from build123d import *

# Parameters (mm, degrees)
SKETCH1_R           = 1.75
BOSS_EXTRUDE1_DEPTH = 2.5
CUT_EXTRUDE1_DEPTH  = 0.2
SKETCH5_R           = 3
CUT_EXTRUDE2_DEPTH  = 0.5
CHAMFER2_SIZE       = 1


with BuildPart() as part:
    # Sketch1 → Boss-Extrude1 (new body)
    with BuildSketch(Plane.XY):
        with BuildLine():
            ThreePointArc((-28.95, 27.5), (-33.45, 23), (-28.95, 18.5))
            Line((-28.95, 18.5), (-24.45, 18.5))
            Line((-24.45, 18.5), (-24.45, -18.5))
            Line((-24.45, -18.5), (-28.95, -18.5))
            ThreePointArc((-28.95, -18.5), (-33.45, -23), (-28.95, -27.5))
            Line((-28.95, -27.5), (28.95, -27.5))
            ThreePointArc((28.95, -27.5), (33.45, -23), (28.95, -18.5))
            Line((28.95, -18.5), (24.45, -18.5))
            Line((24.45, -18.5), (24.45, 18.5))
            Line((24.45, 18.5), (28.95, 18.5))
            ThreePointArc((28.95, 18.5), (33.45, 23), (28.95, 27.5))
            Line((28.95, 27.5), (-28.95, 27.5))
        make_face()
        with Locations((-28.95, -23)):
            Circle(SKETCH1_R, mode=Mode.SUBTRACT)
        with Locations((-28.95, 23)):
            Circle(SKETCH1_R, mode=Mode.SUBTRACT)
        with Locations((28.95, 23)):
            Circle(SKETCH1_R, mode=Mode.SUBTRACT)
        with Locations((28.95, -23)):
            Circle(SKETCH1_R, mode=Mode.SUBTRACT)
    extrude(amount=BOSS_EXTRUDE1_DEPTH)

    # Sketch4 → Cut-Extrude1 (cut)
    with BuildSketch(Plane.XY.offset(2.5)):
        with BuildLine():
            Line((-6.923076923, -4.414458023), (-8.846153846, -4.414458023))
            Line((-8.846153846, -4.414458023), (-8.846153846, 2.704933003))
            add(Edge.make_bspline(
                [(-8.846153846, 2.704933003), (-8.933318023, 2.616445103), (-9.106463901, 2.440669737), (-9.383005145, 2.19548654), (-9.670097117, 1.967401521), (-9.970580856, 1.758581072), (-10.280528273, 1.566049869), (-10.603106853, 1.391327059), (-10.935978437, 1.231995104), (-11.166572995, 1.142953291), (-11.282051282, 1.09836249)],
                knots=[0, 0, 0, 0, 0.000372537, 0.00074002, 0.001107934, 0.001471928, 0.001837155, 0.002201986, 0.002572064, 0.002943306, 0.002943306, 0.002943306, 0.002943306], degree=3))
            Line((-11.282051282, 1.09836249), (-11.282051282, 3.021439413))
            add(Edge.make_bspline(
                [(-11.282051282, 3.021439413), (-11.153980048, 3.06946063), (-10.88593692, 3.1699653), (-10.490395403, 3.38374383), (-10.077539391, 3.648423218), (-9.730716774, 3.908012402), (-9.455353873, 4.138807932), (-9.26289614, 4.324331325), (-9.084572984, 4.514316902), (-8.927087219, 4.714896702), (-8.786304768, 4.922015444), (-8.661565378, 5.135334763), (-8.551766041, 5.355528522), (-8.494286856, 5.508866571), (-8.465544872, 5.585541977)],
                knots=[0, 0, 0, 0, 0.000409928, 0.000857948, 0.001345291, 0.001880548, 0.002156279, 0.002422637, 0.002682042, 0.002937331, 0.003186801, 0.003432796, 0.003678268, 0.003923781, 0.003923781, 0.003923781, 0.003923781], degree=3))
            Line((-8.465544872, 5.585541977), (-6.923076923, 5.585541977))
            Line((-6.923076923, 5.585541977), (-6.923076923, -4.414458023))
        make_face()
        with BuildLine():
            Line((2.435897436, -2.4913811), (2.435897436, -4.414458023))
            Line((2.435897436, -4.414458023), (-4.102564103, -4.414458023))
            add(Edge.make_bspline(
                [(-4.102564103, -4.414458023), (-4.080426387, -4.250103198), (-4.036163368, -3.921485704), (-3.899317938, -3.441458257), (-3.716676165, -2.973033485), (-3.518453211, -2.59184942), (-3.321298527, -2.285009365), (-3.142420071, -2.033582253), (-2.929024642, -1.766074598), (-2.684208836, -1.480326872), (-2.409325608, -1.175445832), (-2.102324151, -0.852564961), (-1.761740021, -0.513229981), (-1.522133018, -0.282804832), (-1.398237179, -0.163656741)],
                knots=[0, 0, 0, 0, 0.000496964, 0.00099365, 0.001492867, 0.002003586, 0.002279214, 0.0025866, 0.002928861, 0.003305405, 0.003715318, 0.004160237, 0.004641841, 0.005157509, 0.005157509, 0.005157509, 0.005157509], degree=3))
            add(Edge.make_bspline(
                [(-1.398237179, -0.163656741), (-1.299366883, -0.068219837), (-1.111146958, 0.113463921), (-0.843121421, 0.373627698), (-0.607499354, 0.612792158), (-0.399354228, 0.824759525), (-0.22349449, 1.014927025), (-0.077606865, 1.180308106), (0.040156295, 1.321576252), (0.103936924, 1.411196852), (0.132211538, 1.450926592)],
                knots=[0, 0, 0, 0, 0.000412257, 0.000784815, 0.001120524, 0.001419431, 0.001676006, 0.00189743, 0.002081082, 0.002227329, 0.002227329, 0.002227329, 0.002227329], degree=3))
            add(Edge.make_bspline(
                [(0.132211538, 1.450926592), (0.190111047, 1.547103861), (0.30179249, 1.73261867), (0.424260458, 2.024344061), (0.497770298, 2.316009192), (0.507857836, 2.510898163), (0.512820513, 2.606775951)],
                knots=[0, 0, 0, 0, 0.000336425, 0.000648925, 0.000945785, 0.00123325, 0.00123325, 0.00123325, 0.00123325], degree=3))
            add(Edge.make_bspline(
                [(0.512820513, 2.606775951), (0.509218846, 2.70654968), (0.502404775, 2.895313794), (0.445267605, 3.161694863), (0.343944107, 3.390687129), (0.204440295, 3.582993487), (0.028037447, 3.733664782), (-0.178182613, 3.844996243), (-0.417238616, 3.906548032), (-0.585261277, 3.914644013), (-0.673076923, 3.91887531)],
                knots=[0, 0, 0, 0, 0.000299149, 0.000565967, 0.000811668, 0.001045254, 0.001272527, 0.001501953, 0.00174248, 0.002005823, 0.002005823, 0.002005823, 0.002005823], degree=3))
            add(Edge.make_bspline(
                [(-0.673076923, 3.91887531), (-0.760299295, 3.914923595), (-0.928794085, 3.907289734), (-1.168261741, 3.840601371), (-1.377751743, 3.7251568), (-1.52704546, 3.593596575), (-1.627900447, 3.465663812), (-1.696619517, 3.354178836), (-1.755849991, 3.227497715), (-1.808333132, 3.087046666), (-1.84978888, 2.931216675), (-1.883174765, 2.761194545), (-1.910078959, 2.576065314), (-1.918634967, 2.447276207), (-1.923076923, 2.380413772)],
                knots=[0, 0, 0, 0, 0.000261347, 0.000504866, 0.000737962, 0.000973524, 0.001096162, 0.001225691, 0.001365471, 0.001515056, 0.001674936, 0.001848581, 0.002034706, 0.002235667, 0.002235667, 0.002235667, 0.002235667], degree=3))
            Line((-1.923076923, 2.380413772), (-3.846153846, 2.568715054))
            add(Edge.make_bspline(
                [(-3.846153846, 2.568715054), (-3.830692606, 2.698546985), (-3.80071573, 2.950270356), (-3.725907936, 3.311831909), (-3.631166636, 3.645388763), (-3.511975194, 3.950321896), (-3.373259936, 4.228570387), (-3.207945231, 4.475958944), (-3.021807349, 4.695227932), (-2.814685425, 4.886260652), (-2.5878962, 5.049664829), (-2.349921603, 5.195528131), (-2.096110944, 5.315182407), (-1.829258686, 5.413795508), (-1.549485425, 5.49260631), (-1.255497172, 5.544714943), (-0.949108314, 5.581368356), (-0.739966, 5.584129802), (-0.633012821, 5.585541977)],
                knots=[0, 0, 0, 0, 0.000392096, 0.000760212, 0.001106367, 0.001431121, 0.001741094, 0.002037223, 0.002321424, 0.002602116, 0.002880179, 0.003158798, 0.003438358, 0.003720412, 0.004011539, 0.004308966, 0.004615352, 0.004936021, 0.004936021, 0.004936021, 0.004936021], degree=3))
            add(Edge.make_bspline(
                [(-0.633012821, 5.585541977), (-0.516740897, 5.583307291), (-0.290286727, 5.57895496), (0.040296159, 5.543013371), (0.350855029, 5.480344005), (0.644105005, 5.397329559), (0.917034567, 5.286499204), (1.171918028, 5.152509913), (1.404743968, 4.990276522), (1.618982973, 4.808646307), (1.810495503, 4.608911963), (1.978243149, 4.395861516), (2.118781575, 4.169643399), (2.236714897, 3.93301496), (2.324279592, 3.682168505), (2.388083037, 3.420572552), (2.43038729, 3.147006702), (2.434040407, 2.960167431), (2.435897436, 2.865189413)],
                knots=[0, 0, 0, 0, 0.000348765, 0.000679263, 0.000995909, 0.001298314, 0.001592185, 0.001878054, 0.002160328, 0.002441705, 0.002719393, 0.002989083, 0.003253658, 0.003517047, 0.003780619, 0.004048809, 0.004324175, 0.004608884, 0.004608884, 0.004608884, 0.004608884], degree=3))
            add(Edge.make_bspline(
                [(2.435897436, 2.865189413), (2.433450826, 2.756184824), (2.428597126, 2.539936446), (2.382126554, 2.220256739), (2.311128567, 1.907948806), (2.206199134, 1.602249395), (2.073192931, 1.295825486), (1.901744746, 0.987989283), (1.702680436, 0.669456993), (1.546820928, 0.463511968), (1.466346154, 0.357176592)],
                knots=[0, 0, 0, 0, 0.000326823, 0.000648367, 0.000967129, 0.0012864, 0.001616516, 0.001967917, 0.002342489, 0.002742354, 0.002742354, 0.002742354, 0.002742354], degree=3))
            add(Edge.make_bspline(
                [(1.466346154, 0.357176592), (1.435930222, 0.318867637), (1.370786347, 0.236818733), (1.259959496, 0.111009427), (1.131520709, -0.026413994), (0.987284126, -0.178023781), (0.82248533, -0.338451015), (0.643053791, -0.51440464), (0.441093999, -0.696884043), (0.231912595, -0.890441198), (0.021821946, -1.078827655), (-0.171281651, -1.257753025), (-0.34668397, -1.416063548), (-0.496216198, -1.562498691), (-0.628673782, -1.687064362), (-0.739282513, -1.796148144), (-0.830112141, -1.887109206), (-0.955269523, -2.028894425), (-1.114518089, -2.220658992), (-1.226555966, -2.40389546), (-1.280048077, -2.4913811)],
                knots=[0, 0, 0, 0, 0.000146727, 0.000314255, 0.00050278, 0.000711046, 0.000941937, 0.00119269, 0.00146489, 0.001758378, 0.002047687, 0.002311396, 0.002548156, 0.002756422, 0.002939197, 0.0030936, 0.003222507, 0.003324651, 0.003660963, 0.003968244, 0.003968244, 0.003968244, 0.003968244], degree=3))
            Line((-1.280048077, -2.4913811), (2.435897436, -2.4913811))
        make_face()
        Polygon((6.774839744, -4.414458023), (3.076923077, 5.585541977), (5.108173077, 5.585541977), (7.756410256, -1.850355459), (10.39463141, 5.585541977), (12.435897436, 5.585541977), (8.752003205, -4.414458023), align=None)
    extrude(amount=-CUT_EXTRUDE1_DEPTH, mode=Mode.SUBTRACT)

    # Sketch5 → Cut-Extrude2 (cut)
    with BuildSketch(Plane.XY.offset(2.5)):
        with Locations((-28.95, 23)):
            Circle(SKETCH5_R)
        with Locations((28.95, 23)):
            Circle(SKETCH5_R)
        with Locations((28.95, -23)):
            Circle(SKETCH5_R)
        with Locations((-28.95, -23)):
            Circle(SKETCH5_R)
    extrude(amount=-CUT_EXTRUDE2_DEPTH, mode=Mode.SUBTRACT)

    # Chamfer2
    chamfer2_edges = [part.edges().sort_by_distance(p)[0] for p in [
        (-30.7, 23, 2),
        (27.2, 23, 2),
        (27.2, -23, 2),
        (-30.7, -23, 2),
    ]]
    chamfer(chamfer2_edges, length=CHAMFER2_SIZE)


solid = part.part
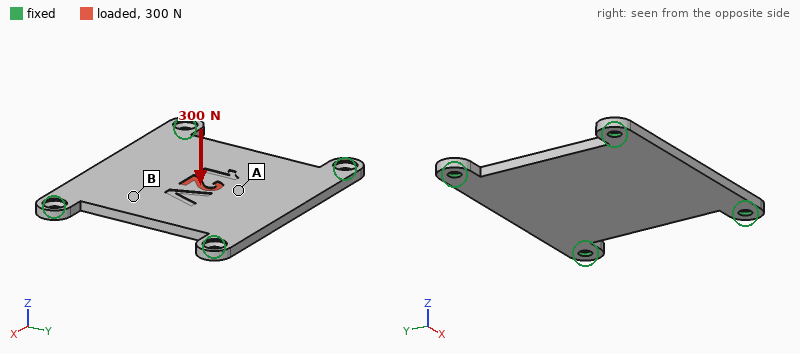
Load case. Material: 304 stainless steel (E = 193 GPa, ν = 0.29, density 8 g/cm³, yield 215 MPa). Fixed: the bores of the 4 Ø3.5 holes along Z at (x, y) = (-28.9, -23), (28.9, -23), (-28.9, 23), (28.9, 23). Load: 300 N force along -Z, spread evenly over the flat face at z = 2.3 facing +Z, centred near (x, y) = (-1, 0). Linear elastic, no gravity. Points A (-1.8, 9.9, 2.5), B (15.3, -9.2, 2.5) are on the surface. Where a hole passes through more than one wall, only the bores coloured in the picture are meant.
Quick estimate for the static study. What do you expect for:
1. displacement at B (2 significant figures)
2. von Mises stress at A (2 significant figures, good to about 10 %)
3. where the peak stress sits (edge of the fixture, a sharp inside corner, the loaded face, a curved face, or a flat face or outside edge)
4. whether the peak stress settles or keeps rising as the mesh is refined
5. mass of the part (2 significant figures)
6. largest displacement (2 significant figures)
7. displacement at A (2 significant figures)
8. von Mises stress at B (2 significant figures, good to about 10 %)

36 µm
47 MPa
edge of the fixture
keeps rising
58 g
62 µm
53 µm
21 MPa
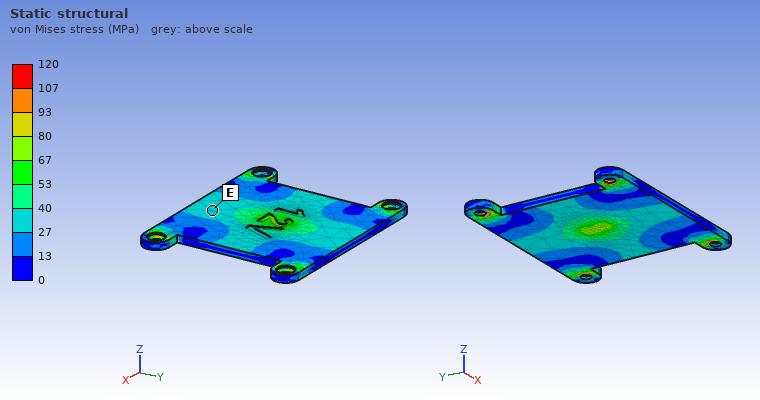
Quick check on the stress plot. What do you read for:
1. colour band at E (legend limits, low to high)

27 to 40 MPa
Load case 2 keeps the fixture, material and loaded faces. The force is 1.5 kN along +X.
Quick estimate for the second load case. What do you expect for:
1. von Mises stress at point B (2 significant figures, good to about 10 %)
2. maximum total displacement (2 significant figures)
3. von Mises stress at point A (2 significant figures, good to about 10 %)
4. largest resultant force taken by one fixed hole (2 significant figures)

13 MPa
5.9 µm
27 MPa
400 N
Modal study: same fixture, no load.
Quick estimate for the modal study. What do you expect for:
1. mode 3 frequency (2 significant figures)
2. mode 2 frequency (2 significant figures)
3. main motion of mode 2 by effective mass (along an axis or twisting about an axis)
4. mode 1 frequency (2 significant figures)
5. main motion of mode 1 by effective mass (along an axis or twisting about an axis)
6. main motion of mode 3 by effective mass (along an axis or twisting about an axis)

5200 Hz
3900 Hz
twisting about X
2400 Hz
along Z
twisting about Y
